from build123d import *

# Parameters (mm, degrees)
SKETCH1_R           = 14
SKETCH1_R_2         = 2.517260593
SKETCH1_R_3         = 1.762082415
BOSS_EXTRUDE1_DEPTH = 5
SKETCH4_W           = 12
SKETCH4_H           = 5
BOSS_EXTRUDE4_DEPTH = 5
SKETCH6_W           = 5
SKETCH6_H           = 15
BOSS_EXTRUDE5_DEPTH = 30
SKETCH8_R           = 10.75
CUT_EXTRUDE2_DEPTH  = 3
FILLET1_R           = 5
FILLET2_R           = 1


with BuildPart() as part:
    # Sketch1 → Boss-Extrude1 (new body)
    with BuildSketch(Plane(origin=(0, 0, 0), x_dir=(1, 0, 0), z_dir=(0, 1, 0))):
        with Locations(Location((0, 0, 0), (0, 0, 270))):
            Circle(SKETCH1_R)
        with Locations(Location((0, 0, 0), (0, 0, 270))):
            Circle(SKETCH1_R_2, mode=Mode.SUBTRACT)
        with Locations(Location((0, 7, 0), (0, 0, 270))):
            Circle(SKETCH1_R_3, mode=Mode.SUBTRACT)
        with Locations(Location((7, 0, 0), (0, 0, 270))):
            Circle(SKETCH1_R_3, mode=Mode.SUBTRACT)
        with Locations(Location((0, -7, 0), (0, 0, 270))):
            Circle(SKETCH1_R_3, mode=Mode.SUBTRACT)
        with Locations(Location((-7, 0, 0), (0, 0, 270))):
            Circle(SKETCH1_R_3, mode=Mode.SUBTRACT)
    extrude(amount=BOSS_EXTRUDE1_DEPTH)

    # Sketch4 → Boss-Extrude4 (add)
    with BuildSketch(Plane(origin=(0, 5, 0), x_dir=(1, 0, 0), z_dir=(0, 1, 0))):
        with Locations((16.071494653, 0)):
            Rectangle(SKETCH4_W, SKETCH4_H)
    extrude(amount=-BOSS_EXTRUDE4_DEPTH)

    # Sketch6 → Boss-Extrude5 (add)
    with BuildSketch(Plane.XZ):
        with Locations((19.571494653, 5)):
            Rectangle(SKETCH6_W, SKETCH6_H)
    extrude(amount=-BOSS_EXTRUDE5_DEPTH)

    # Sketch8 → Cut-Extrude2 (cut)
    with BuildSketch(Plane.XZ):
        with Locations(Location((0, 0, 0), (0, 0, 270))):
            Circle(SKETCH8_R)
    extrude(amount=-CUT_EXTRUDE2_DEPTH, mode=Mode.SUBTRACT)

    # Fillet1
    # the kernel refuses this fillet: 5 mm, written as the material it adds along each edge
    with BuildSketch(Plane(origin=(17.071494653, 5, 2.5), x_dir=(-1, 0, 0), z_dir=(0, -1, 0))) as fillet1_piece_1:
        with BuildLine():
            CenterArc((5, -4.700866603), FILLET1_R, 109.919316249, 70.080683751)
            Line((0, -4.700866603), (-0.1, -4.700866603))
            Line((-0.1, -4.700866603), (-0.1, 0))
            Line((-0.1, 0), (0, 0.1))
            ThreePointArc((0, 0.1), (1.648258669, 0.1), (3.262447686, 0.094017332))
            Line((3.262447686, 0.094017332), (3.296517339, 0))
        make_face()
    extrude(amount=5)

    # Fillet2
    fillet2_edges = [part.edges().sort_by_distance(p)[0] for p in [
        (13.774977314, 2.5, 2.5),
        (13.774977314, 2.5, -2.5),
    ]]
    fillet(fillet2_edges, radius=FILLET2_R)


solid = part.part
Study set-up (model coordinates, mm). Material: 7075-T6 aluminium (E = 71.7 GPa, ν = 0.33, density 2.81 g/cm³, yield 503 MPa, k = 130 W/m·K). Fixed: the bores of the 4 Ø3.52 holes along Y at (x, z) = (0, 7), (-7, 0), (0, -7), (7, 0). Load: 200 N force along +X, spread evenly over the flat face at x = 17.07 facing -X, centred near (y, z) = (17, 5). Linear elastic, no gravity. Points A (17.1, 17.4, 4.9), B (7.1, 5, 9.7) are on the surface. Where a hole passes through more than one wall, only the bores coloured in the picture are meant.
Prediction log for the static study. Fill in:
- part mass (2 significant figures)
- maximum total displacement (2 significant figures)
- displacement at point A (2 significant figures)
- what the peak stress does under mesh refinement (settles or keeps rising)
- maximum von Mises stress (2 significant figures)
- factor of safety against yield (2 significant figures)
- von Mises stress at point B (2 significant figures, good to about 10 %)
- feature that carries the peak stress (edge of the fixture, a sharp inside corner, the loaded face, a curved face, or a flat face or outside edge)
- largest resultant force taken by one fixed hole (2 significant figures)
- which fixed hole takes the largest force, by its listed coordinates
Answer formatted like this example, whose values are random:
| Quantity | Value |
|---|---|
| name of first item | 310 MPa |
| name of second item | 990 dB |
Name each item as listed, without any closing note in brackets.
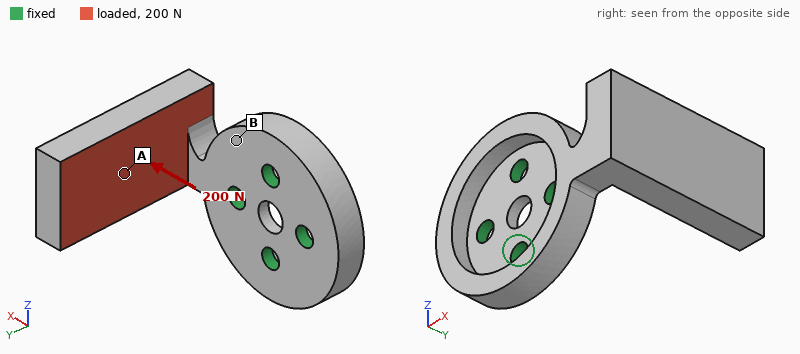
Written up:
| Quantity | Value |
|---|---|
| part mass | 12 g |
| maximum total displacement | 0.36 mm |
| displacement at point A | 0.18 mm |
| what the peak stress does under mesh refinement | settles |
| maximum von Mises stress | 330 MPa |
| factor of safety against yield | 1.5 |
| von Mises stress at point B | 34 MPa |
| feature that carries the peak stress | a curved face |
| largest resultant force taken by one fixed hole | 410 N |
| which fixed hole takes the largest force, by its listed coordinates | (7, 0) |
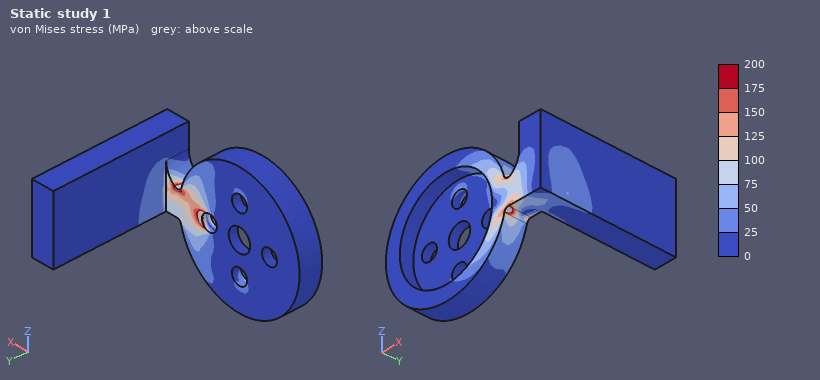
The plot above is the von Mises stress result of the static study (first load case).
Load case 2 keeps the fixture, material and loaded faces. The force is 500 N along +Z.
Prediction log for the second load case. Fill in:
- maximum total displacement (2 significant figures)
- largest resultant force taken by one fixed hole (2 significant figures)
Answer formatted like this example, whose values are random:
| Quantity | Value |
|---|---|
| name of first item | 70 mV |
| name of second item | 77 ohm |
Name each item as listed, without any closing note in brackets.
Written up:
| Quantity | Value |
|---|---|
| maximum total displacement | 0.60 mm |
| largest resultant force taken by one fixed hole | 380 N |
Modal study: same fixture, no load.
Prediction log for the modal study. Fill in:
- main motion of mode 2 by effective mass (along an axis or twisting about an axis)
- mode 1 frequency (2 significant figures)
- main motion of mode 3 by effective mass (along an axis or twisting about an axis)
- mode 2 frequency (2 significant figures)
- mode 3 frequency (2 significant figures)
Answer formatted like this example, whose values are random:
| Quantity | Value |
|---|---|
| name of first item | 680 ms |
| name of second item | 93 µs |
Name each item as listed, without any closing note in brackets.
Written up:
| Quantity | Value |
|---|---|
| main motion of mode 2 by effective mass | along Z |
| mode 1 frequency | 1800 Hz |
| main motion of mode 3 by effective mass | along Y |
| mode 2 frequency | 2300 Hz |
| mode 3 frequency | 7000 Hz |
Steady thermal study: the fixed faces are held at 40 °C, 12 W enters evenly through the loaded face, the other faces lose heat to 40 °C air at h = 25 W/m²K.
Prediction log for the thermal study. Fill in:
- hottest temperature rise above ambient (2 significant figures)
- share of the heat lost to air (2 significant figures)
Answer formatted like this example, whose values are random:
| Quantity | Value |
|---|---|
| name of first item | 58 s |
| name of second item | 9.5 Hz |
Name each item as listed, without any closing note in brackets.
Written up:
| Quantity | Value |
|---|---|
| hottest temperature rise above ambient | 47 K |
| share of the heat lost to air | 8.9 % |
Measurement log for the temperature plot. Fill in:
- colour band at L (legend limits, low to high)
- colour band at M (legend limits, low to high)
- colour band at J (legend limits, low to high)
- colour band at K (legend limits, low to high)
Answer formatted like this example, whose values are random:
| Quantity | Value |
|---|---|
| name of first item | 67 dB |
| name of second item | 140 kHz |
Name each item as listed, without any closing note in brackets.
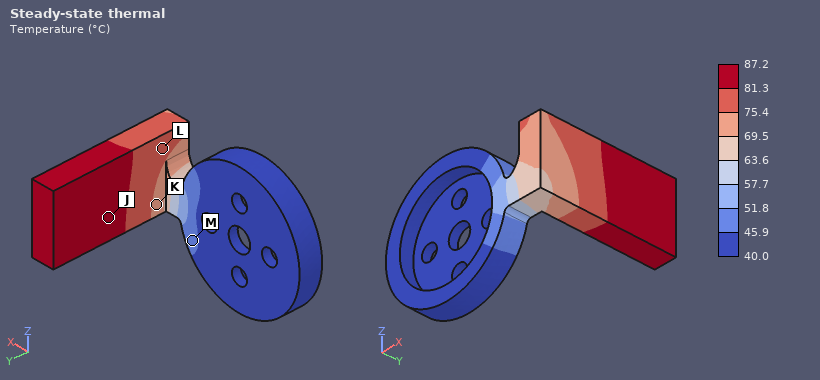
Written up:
| Quantity | Value |
|---|---|
| colour band at L | 75.4 to 81.3 °C |
| colour band at M | 45.9 to 51.8 °C |
| colour band at J | 81.3 to 87.2 °C |
| colour band at K | 69.5 to 75.4 °C |
